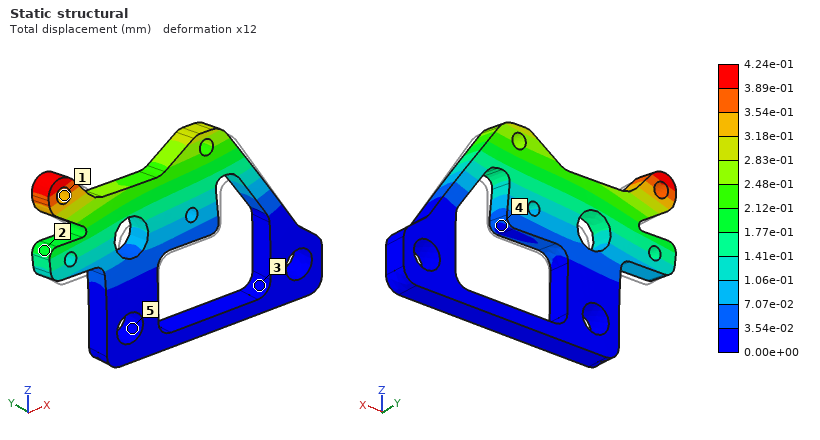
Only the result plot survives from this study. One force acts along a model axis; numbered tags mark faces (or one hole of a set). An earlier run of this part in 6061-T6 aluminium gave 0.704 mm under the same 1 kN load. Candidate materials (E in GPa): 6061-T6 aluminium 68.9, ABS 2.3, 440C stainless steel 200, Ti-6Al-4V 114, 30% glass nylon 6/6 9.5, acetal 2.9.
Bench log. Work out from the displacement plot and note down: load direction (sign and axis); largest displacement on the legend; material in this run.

+Y
4.24e-01 mm
Ti-6Al-4V
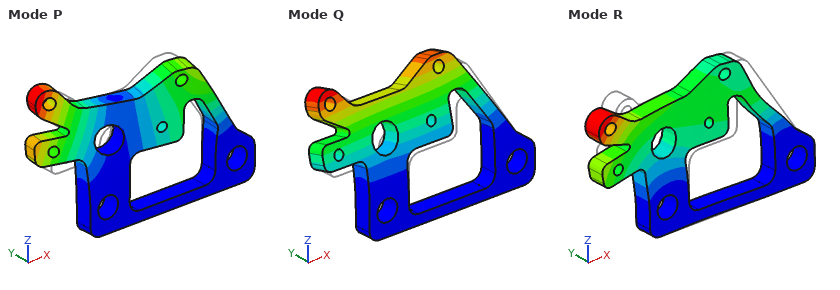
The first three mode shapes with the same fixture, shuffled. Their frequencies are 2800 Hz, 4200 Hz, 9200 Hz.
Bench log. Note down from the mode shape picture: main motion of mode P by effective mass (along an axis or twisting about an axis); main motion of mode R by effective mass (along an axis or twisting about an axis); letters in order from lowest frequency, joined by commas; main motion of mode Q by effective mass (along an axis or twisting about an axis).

twisting about Z
along X
Q, P, R
along Y
